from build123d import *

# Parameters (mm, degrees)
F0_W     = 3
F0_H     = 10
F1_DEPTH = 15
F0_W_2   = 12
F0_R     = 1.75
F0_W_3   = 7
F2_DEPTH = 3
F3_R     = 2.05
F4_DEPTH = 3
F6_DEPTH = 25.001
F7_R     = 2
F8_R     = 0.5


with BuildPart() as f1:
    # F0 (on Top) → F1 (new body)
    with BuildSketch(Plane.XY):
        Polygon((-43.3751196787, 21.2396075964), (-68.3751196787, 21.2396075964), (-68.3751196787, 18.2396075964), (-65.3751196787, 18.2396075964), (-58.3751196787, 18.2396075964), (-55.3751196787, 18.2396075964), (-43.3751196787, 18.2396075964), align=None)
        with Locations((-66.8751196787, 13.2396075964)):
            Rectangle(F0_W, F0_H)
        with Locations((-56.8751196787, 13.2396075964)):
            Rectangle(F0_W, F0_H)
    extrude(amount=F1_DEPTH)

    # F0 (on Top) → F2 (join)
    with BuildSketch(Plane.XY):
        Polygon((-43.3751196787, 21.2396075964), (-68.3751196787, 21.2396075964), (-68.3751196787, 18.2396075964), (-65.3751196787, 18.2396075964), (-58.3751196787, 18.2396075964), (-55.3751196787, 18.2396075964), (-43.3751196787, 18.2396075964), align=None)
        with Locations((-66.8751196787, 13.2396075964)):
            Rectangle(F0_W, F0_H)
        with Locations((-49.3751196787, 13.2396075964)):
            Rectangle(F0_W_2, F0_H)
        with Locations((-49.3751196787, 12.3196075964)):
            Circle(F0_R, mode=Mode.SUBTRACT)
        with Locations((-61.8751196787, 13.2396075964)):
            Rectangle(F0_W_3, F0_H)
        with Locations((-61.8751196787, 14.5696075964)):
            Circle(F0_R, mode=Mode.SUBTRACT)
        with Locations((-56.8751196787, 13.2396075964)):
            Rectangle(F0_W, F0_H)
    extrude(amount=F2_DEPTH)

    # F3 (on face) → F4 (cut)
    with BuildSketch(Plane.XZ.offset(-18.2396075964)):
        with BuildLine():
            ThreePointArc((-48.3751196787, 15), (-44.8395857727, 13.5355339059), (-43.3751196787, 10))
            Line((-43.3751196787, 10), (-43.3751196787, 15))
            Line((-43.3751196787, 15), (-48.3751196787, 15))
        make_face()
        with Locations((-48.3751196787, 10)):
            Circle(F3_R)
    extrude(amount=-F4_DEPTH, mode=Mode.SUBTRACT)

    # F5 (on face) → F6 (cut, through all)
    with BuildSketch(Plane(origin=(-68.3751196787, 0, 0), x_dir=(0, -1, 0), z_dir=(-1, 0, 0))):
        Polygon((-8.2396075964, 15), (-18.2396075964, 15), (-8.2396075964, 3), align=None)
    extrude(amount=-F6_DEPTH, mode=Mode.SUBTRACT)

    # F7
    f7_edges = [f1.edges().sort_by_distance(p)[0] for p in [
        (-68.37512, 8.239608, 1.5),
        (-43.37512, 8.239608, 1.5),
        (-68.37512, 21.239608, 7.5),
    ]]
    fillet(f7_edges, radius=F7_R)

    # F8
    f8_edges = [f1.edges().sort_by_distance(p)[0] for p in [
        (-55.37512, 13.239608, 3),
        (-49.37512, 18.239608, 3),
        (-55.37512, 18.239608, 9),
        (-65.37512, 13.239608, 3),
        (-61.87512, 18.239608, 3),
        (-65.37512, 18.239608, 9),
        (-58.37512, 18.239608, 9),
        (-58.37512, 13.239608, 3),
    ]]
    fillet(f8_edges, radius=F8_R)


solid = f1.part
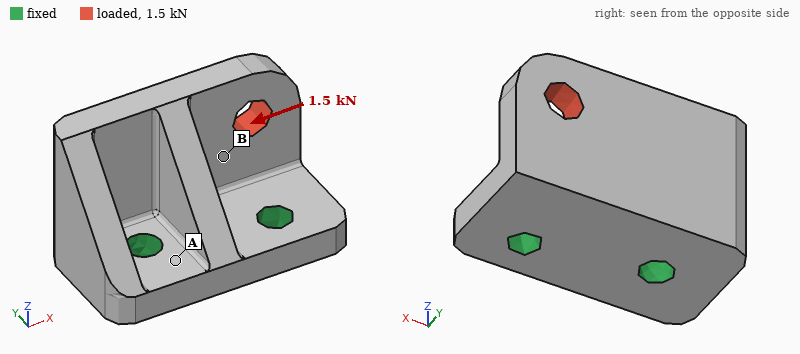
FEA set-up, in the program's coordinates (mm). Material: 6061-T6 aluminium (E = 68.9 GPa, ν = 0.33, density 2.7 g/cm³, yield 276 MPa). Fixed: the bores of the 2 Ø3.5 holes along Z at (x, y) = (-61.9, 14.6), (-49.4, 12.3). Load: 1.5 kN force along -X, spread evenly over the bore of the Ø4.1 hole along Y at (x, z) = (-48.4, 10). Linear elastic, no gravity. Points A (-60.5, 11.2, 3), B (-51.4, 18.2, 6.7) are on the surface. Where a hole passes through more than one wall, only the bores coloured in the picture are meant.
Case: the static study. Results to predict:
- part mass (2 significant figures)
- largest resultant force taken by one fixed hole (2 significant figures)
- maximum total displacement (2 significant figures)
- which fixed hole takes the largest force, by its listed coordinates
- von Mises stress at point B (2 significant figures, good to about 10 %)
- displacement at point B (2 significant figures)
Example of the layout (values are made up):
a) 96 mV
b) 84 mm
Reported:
a) 5.7 g
b) 1.4 kN
c) 58 µm
d) (-61.9, 14.6)
e) 82 MPa
f) 26 µm
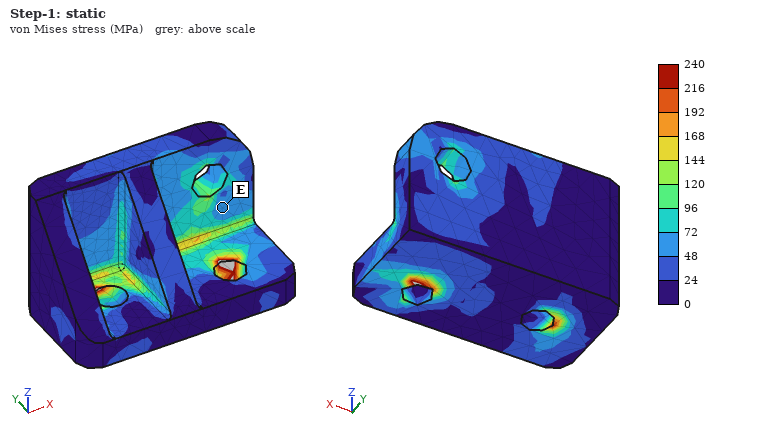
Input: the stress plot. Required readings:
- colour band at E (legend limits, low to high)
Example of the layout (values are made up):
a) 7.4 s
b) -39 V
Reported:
a) 48 to 72 MPa
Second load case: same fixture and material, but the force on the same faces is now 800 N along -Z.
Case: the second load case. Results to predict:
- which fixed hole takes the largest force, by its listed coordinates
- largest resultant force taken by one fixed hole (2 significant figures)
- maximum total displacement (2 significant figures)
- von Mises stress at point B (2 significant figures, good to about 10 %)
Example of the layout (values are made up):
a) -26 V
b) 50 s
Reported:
a) (-49.4, 12.3)
b) 710 N
c) 61 µm
d) 41 MPa
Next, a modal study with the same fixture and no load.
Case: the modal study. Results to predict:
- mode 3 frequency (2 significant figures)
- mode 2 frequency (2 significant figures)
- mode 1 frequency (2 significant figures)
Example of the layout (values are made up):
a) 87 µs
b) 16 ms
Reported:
a) 25 kHz
b) 18 kHz
c) 13 kHz
